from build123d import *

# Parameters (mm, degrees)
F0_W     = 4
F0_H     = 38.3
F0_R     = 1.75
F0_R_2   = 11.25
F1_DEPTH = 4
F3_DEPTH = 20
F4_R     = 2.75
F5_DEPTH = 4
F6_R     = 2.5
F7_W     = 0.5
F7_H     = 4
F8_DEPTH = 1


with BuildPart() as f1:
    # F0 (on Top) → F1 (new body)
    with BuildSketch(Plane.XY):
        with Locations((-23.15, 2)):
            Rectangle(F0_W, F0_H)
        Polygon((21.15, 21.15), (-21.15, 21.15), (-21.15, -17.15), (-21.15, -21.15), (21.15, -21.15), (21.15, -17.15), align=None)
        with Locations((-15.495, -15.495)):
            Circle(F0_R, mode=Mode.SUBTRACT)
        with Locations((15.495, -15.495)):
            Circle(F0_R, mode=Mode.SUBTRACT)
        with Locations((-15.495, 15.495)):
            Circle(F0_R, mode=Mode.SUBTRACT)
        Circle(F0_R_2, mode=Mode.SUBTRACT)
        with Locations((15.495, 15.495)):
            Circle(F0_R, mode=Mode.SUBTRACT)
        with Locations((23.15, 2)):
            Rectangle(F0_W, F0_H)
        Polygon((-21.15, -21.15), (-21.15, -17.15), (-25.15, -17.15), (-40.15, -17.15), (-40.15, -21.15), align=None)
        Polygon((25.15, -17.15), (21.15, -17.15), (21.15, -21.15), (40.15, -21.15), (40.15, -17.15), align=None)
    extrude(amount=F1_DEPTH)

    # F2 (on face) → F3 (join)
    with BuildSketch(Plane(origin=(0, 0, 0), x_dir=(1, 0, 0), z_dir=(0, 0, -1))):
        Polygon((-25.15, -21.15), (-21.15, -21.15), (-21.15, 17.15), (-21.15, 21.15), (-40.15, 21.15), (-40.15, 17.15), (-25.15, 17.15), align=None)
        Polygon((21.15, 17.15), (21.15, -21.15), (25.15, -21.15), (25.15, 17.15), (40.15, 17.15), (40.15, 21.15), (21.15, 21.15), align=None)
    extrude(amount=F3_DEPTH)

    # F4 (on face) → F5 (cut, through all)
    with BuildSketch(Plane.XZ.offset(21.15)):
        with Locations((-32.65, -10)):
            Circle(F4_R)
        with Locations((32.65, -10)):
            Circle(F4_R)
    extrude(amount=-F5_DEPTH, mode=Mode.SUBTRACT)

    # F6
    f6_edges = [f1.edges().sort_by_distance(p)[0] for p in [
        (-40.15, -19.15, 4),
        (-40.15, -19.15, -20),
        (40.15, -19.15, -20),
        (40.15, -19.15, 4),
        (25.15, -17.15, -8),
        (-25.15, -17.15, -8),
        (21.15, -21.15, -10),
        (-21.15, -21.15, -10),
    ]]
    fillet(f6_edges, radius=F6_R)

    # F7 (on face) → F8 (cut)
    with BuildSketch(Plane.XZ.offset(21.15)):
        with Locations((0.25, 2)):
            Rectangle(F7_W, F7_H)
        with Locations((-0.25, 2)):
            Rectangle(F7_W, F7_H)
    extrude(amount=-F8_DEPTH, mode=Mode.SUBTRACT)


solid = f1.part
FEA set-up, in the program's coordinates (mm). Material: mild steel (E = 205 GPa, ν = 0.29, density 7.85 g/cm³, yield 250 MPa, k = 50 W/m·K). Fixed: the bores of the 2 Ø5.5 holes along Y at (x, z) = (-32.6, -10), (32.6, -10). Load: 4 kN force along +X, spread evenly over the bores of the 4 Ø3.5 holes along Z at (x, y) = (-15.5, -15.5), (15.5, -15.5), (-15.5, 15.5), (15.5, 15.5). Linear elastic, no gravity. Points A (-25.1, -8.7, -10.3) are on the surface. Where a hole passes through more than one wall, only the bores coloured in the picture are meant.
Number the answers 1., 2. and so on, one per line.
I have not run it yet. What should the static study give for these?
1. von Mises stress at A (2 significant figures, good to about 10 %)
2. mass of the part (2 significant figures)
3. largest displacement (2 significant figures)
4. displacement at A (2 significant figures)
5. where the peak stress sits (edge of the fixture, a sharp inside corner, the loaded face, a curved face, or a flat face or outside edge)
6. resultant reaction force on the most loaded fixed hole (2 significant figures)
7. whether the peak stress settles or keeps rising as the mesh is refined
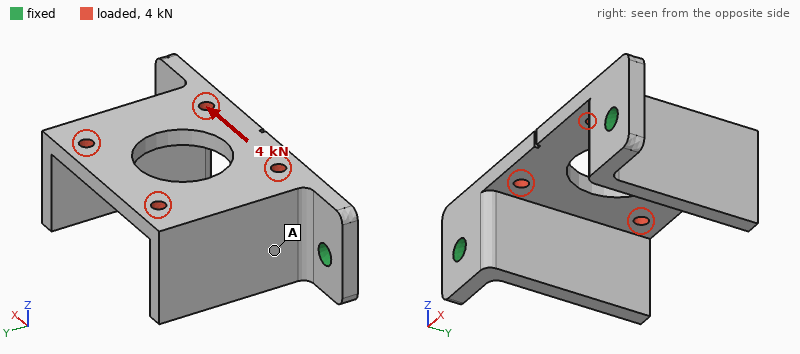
1. 26 MPa
2. 130 g
3. 76 µm
4. 18 µm
5. edge of the fixture
6. 2.4 kN
7. keeps rising
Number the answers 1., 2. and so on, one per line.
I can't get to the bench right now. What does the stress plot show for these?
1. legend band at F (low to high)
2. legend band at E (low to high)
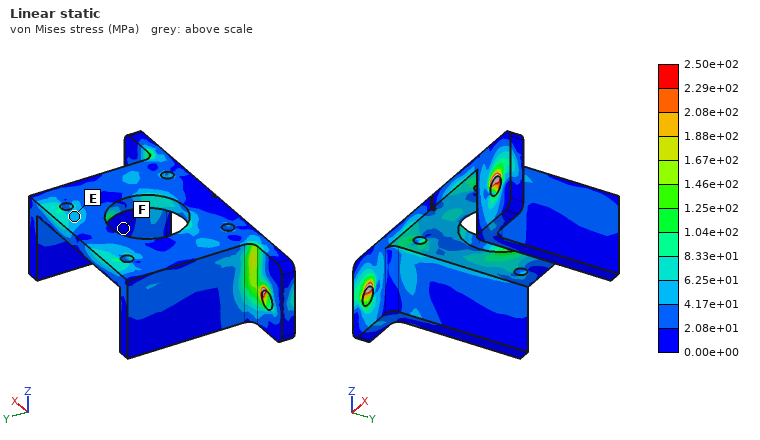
1. 0.00e+00 to 2.08e+01 MPa
2. 4.17e+01 to 6.25e+01 MPa
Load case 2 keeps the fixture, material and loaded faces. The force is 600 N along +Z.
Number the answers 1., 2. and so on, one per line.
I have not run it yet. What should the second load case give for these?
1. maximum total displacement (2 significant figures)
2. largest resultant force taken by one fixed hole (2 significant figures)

1. 47 µm
2. 330 N
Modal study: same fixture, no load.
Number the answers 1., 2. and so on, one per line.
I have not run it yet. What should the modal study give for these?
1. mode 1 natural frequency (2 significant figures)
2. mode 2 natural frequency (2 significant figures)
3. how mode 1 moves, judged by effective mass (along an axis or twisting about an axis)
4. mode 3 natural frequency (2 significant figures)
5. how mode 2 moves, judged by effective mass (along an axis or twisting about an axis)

1. 2200 Hz
2. 2800 Hz
3. along Z
4. 4800 Hz
5. along X
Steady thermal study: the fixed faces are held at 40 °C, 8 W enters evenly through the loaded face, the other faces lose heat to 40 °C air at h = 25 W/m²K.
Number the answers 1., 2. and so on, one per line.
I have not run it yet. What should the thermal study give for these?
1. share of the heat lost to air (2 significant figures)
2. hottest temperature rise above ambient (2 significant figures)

1. 31 %
2. 19 K
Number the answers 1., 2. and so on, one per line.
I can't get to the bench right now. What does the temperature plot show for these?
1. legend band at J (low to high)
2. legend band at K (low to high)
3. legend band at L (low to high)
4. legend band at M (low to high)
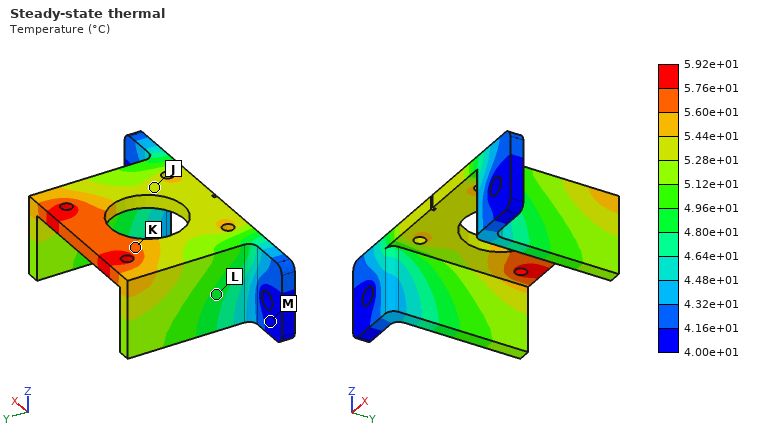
1. 5.28e+01 to 5.44e+01 °C
2. 5.60e+01 to 5.76e+01 °C
3. 4.80e+01 to 4.96e+01 °C
4. 4.00e+01 to 4.16e+01 °C
